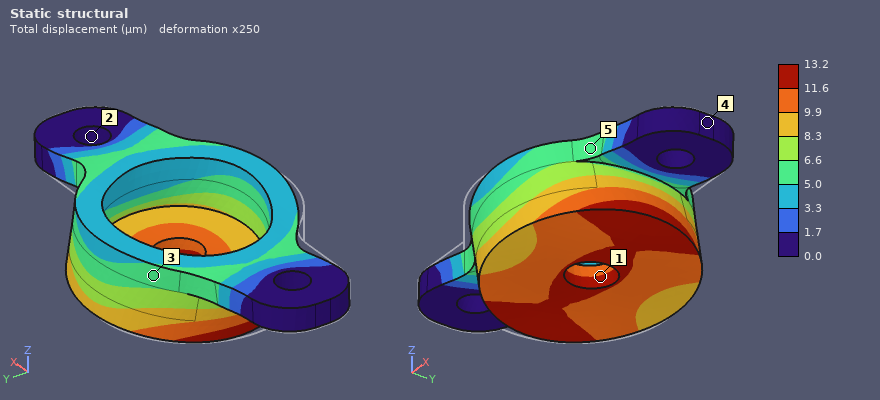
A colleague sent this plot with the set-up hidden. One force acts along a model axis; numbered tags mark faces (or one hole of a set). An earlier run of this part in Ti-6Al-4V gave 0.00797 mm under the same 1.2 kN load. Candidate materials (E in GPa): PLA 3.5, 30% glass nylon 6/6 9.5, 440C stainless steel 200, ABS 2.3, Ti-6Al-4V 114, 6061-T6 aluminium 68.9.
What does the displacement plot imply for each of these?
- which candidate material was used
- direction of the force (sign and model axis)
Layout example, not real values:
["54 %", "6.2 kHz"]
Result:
["6061-T6 aluminium", "+X"]
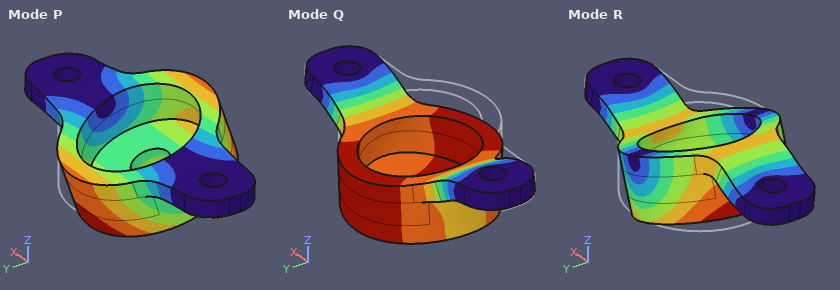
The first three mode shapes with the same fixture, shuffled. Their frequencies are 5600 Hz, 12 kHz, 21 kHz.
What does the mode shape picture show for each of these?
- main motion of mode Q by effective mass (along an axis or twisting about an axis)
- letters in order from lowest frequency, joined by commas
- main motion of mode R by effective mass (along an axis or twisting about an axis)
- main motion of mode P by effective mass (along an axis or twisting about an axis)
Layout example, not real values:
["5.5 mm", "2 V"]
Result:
["along Z", "P, Q, R", "along X", "along Y"]
